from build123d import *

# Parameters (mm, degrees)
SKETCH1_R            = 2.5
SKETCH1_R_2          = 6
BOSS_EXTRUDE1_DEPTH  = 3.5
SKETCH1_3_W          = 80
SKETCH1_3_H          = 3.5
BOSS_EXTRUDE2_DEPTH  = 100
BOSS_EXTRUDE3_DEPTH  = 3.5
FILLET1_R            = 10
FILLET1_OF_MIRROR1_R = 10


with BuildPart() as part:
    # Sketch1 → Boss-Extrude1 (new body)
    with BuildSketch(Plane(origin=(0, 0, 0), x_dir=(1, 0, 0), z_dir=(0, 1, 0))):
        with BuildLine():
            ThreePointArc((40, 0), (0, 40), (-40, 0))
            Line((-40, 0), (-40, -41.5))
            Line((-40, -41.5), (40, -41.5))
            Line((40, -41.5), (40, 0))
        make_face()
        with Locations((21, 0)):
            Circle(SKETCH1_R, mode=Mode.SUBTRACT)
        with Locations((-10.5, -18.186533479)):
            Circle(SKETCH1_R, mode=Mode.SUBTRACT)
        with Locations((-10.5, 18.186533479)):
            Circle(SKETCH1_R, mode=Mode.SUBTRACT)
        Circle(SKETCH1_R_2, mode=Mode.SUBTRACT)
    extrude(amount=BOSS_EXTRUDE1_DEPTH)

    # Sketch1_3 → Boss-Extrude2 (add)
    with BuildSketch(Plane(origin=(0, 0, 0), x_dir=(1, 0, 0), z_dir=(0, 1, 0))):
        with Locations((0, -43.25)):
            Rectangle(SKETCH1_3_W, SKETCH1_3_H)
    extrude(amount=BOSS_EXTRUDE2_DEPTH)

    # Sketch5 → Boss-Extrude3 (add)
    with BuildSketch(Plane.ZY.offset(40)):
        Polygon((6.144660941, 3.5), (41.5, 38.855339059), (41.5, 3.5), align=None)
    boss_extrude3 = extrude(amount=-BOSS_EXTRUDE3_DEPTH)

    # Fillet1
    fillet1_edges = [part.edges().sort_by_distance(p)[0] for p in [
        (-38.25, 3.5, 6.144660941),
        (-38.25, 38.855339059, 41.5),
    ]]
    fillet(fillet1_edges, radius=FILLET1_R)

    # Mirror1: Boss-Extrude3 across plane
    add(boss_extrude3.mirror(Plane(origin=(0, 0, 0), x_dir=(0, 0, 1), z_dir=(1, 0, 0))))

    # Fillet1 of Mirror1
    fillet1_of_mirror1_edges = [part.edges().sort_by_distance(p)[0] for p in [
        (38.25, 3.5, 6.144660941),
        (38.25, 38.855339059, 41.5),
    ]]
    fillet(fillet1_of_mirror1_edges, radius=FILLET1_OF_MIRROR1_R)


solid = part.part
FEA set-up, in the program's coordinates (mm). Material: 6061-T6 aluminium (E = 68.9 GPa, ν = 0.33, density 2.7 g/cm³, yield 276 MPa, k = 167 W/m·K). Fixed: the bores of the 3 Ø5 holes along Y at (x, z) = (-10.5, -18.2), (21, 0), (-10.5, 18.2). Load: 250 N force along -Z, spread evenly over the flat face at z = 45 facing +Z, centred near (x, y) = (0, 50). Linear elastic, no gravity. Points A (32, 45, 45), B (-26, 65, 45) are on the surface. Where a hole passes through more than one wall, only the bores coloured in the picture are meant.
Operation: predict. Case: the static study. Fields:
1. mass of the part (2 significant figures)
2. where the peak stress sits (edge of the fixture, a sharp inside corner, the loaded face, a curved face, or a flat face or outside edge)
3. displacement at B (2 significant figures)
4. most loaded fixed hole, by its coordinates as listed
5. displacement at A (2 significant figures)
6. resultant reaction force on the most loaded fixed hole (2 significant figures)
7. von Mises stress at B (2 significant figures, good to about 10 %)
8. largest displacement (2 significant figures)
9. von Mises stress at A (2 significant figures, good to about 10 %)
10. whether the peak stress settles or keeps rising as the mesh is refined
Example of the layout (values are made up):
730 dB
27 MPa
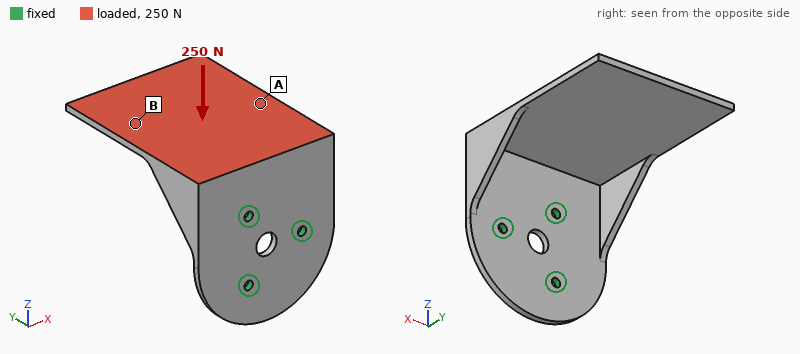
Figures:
140 g
edge of the fixture
0.56 mm
(-10.5, 18.2)
0.38 mm
250 N
15 MPa
1.1 mm
32 MPa
keeps rising
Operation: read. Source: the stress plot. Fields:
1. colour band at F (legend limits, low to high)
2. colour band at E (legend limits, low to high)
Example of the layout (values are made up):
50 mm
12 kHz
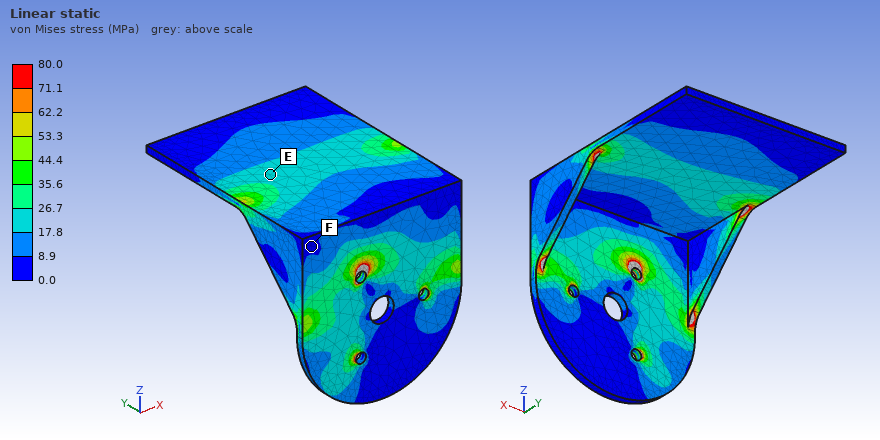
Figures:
0.0 to 8.9 MPa
17.8 to 26.7 MPa
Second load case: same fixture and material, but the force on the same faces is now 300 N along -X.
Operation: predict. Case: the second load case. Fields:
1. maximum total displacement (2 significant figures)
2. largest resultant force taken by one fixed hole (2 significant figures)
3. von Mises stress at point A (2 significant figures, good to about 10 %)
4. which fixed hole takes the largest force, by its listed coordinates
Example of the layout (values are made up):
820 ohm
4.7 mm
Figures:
0.76 mm
400 N
14 MPa
(-10.5, 18.2)
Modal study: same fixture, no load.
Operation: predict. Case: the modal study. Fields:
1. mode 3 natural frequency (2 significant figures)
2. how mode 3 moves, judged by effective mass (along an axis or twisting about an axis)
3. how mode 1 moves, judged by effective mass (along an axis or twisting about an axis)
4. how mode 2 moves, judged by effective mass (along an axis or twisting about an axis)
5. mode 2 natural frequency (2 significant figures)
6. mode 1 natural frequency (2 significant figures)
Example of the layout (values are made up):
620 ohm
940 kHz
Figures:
1100 Hz
along Y
along Z
along X
460 Hz
330 Hz
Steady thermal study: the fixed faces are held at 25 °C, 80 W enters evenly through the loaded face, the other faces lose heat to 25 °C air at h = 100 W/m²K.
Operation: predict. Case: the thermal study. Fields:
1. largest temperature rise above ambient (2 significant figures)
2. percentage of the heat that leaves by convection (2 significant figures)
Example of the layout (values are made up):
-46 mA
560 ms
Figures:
52 K
63 %
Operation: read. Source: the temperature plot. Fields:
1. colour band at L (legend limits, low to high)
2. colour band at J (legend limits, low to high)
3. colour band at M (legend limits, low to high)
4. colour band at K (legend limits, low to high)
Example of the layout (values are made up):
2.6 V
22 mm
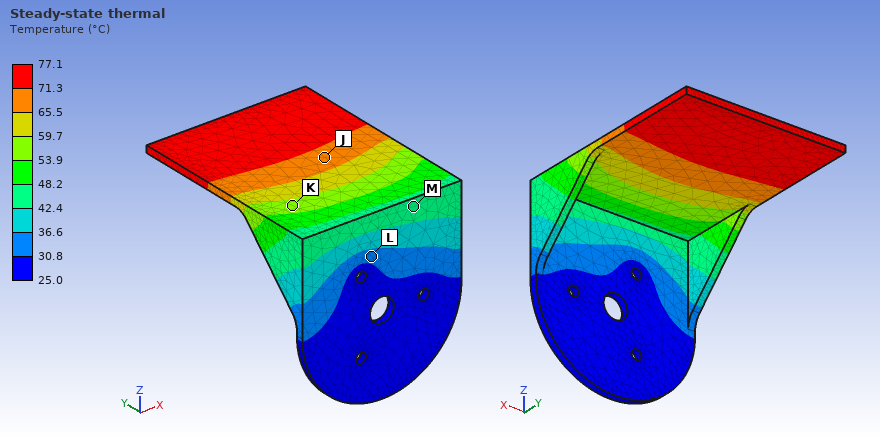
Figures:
30.8 to 36.6 °C
65.5 to 71.3 °C
42.4 to 48.2 °C
53.9 to 59.7 °C
